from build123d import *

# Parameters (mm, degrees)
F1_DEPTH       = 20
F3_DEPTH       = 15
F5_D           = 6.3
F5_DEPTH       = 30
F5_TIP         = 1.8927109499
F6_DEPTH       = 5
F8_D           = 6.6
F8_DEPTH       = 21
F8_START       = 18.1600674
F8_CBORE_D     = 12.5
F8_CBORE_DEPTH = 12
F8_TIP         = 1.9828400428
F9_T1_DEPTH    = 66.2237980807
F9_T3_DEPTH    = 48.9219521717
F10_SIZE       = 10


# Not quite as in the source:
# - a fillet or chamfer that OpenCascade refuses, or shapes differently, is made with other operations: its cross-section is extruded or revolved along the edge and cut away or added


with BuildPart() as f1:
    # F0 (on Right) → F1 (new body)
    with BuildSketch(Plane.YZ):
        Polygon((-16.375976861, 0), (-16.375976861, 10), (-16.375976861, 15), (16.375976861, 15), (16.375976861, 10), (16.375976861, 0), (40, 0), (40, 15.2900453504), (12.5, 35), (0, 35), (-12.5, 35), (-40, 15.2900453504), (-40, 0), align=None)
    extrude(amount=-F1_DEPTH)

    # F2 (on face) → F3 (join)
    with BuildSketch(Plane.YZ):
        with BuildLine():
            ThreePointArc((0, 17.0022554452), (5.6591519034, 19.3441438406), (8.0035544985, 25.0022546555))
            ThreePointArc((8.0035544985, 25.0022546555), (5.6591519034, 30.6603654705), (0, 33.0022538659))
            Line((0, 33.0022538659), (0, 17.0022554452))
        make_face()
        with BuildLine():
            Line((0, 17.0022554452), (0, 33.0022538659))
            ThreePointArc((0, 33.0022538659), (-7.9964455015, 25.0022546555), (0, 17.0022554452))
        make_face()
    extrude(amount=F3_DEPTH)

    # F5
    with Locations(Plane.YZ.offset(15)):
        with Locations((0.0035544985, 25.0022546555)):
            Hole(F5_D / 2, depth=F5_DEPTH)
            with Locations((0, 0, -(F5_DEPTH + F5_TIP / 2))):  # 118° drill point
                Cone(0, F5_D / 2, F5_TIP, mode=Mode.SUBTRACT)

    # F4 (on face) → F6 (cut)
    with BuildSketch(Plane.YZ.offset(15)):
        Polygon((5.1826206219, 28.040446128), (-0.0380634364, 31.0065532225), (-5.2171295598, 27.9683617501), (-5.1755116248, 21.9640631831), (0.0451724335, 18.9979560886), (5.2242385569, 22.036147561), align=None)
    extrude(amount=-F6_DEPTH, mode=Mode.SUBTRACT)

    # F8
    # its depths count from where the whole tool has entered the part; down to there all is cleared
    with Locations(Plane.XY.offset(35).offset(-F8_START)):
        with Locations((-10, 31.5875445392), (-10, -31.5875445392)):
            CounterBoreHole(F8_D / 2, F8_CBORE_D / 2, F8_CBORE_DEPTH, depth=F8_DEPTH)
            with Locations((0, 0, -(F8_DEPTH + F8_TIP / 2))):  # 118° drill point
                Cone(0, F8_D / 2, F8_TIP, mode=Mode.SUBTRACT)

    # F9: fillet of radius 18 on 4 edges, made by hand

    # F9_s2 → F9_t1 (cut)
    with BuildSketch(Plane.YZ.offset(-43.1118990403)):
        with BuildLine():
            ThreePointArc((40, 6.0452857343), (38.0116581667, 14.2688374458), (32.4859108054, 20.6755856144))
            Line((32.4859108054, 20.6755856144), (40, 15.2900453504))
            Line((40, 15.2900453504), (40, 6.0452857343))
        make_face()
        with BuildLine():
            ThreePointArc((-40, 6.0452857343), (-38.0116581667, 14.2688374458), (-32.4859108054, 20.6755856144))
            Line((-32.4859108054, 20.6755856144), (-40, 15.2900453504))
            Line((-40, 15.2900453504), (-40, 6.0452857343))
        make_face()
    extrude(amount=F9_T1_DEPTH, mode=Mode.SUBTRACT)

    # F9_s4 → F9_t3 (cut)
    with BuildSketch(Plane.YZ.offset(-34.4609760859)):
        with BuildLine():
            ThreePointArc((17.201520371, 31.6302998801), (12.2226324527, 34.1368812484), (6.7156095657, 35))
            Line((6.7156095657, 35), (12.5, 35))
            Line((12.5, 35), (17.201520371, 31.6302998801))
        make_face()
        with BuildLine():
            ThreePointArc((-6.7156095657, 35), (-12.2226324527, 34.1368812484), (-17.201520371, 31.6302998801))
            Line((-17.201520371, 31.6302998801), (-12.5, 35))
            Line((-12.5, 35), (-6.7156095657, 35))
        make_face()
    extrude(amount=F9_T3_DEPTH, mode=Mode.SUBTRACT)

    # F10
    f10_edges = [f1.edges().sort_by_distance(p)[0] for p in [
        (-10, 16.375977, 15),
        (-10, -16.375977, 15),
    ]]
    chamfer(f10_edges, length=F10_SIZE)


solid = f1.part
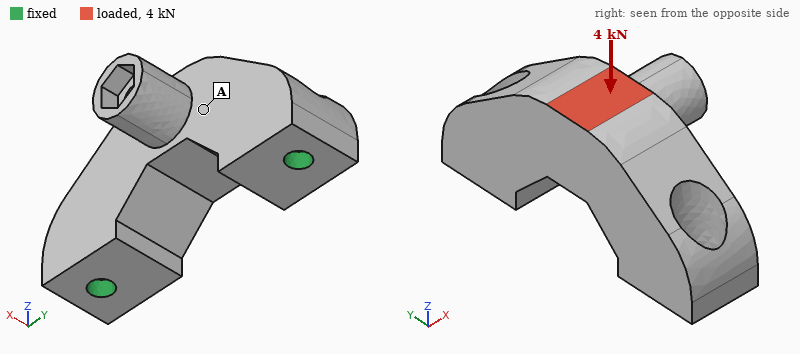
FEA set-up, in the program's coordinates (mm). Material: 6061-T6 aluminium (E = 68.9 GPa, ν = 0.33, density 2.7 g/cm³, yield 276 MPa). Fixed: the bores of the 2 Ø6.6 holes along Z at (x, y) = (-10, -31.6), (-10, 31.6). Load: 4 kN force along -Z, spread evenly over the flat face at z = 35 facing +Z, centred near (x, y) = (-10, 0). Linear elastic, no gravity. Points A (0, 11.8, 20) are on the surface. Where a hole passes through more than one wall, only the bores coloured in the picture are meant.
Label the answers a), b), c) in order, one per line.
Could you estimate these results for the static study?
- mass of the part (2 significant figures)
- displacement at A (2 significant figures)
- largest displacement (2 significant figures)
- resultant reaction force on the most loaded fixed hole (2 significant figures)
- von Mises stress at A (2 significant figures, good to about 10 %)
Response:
a) 92 g
b) 9.5 µm
c) 14 µm
d) 2.6 kN
e) 11 MPa
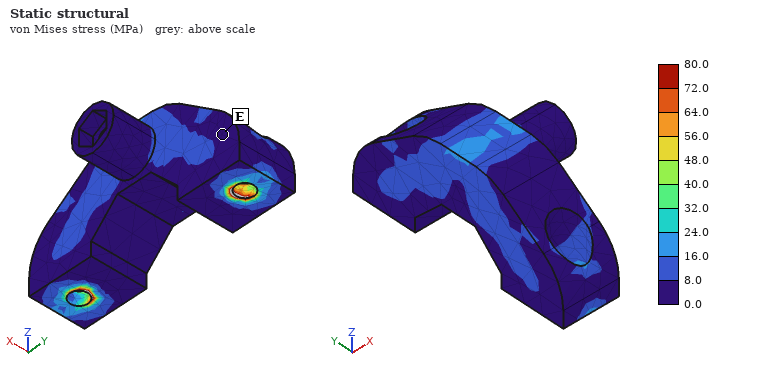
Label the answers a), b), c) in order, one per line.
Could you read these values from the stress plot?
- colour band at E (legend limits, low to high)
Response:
a) 0.0 to 8.0 MPa
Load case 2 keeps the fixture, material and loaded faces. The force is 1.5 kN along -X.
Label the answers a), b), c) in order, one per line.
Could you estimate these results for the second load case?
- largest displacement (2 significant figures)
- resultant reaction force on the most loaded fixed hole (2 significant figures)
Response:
a) 0.12 mm
b) 750 N
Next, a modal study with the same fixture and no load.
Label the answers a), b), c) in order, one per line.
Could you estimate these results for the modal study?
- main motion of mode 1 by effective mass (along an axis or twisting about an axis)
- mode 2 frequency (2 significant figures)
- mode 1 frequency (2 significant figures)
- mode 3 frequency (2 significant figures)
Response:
a) along X
b) 12 kHz
c) 3500 Hz
d) 12 kHz
